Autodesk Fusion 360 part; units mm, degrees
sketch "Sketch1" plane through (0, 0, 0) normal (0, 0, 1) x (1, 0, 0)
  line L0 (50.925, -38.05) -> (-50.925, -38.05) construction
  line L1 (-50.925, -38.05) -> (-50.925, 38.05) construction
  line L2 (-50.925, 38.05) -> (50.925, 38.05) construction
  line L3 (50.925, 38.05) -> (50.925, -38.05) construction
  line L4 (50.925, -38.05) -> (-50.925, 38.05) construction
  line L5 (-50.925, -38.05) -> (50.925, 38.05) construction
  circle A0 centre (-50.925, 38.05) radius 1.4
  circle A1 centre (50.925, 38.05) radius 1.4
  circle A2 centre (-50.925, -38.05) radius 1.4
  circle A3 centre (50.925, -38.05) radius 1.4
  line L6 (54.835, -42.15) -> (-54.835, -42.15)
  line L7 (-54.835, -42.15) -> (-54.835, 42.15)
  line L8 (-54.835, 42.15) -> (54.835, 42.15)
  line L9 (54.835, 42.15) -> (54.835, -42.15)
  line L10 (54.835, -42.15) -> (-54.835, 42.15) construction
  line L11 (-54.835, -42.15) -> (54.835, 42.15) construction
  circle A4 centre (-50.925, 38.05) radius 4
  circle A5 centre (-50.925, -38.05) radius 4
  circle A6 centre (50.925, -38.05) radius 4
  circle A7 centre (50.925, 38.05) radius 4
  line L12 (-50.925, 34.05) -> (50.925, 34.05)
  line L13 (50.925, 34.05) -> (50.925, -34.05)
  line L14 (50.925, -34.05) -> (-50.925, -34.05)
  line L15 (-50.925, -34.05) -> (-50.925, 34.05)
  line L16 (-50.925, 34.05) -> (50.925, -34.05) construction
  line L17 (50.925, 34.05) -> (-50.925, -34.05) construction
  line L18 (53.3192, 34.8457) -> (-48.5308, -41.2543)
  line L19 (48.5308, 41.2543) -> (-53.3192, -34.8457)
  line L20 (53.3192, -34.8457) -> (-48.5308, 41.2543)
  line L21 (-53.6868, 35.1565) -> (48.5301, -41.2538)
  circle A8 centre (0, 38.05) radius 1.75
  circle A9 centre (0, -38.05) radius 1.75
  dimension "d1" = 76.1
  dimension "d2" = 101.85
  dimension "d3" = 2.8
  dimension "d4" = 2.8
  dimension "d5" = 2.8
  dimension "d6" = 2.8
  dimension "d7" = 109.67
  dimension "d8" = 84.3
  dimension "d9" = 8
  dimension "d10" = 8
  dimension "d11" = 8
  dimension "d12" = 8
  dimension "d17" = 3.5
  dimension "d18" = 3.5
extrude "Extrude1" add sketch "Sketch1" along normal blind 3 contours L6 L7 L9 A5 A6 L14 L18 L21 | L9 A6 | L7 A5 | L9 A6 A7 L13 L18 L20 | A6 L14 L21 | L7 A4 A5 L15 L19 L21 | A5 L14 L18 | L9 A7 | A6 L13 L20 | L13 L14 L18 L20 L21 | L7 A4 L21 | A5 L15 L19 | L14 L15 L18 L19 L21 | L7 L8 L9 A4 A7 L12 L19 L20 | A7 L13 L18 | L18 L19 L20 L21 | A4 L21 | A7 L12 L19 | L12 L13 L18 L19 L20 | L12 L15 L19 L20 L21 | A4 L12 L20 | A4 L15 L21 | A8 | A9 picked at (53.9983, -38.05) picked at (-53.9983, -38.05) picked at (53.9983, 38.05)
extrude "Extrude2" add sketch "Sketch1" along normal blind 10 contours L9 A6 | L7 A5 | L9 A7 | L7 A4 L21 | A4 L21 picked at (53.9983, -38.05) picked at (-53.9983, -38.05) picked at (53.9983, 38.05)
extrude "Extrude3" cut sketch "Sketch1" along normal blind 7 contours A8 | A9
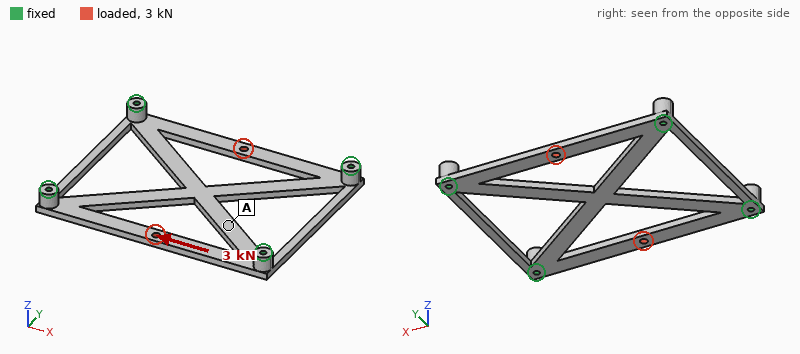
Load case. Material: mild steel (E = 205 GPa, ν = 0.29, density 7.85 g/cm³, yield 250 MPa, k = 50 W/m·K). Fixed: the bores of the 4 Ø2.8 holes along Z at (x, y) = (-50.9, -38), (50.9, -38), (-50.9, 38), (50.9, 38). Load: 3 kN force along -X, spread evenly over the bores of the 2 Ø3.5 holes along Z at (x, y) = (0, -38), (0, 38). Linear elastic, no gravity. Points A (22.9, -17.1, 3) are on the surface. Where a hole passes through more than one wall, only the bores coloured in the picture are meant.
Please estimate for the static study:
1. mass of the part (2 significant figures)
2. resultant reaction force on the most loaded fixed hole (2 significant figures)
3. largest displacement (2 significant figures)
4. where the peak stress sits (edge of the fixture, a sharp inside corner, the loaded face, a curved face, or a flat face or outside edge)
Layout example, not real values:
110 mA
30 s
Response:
100 g
750 N
7.7 µm
the loaded face
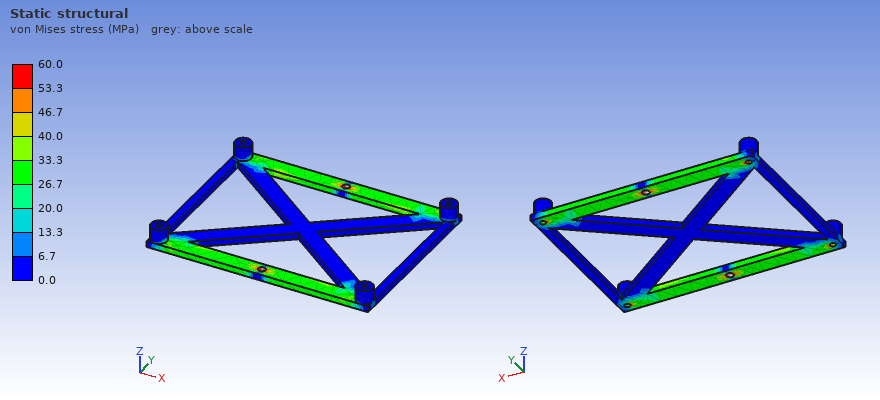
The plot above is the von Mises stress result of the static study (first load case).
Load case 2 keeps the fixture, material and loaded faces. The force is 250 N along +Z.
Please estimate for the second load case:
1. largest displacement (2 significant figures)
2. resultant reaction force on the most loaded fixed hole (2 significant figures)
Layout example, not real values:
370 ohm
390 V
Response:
0.16 mm
67 N
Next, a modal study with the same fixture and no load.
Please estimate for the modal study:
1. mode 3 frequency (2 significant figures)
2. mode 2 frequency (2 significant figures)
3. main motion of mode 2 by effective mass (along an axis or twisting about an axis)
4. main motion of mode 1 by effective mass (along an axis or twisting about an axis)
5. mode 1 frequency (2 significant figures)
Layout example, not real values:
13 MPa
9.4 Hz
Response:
1900 Hz
1800 Hz
twisting about X
along Z
1200 Hz
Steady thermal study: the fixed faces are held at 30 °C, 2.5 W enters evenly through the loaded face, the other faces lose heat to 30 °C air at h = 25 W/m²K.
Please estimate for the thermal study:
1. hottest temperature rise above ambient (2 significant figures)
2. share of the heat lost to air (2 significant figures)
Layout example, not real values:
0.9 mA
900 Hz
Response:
18 K
41 %
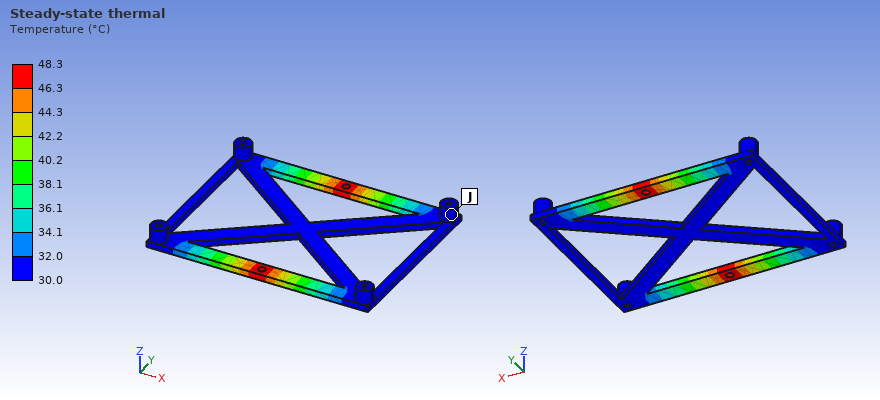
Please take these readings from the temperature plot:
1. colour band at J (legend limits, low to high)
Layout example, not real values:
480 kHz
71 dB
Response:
30.0 to 32.0 °C
